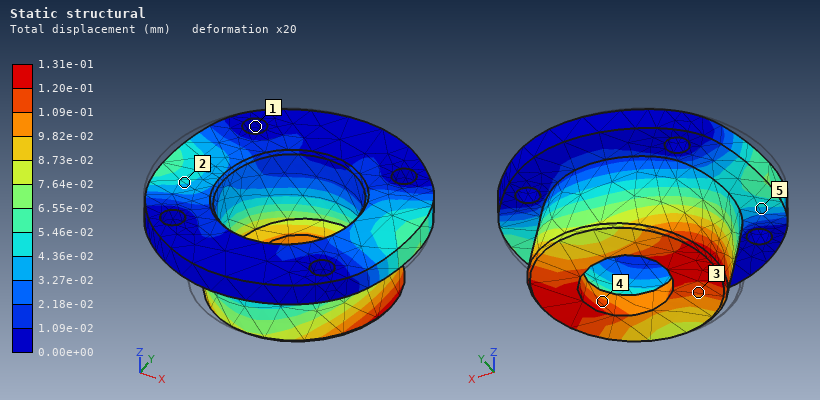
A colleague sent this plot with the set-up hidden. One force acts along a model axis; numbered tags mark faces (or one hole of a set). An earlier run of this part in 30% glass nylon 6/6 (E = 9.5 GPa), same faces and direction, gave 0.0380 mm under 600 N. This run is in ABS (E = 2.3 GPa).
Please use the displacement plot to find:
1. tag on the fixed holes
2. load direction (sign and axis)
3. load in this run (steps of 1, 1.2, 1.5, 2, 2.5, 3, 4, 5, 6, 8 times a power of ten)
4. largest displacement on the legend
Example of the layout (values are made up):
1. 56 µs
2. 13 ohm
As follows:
1. 1
2. +X
3. 500 N
4. 1.31e-01 mm
